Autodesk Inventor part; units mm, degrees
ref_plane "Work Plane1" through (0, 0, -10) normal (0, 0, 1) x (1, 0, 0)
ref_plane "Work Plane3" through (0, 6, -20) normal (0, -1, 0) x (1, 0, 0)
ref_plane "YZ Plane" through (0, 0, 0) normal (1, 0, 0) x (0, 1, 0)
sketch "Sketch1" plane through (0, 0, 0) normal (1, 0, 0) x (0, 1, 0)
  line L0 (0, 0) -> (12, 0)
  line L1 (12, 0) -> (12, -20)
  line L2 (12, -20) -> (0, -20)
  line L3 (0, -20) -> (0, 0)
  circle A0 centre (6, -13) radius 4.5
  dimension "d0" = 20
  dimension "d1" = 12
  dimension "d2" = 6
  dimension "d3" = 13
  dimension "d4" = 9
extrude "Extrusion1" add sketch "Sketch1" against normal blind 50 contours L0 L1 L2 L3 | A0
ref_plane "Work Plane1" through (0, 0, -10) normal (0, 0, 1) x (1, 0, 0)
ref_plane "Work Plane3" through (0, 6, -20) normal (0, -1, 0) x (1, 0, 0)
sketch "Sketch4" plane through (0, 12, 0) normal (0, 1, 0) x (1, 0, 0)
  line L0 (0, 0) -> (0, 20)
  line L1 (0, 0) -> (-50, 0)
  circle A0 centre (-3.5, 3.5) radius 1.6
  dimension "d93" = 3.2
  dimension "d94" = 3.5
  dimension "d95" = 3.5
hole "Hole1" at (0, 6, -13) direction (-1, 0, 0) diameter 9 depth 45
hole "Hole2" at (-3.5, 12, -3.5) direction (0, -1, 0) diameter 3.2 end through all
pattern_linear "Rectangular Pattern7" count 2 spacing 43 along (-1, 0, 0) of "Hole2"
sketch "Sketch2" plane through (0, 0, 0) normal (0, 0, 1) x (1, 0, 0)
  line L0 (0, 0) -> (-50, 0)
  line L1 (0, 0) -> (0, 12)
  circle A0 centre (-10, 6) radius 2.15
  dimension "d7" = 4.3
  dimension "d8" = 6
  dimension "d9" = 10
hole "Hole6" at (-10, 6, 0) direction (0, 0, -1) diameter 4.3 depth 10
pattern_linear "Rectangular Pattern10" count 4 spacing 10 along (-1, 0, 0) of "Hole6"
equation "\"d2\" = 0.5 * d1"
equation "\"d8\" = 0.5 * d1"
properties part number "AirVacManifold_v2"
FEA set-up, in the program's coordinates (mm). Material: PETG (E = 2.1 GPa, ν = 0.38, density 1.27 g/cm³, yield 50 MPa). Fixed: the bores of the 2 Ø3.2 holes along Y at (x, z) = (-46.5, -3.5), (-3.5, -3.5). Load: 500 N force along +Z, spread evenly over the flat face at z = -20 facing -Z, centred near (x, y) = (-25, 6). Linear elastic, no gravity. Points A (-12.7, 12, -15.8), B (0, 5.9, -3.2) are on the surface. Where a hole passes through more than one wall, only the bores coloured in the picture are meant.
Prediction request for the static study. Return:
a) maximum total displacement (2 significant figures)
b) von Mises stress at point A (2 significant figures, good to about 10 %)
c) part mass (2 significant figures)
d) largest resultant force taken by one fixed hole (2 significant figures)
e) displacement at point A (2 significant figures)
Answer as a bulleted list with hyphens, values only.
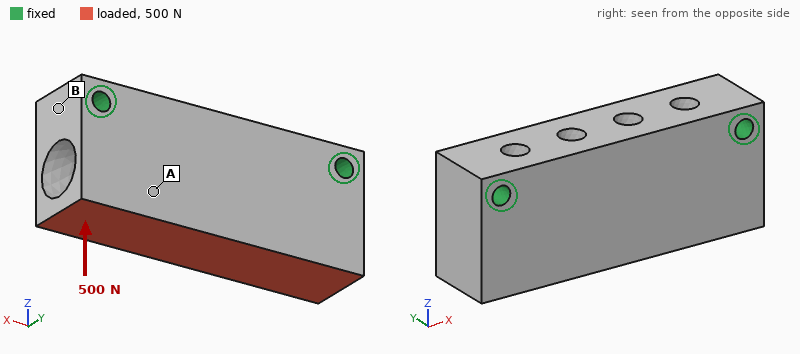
- 69 µm
- 2.8 MPa
- 11 g
- 270 N
- 39 µm
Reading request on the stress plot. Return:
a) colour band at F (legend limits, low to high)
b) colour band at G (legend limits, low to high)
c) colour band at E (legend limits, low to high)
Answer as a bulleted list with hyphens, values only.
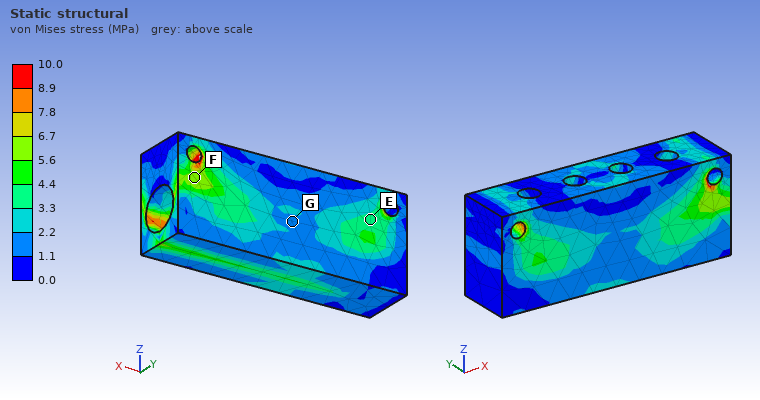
- 5.6 to 6.7 MPa
- 1.1 to 2.2 MPa
- 3.3 to 4.4 MPa
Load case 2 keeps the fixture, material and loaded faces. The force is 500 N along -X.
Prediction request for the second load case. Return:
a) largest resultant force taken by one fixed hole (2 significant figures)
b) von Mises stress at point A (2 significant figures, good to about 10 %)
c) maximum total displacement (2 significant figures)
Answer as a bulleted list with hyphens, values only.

- 310 N
- 5.0 MPa
- 85 µm
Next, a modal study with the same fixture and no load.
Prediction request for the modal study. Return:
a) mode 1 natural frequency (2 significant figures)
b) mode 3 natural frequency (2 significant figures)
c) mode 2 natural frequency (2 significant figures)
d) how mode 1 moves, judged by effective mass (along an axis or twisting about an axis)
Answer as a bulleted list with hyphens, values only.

- 3400 Hz
- 5600 Hz
- 5500 Hz
- along Y
